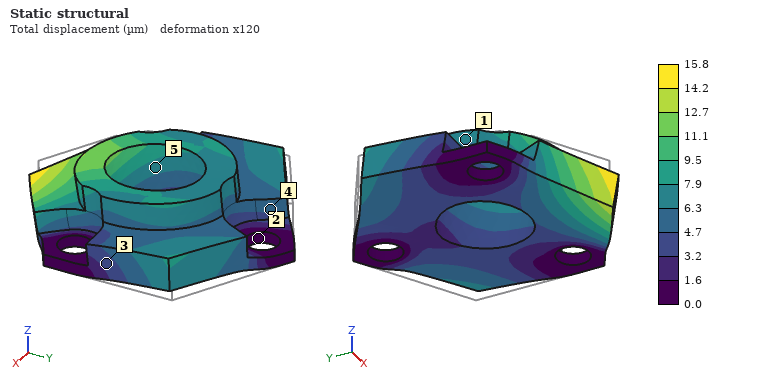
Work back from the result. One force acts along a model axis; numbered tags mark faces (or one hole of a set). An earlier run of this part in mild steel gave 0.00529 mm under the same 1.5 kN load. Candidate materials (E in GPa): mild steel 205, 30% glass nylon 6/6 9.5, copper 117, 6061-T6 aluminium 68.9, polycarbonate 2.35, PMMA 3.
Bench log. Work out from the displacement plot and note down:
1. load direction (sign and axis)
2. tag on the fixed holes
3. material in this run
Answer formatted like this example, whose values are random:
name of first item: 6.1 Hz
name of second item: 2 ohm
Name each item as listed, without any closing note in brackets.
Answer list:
load direction: -Y
tag on the fixed holes: 2
material in this run: 6061-T6 aluminium
